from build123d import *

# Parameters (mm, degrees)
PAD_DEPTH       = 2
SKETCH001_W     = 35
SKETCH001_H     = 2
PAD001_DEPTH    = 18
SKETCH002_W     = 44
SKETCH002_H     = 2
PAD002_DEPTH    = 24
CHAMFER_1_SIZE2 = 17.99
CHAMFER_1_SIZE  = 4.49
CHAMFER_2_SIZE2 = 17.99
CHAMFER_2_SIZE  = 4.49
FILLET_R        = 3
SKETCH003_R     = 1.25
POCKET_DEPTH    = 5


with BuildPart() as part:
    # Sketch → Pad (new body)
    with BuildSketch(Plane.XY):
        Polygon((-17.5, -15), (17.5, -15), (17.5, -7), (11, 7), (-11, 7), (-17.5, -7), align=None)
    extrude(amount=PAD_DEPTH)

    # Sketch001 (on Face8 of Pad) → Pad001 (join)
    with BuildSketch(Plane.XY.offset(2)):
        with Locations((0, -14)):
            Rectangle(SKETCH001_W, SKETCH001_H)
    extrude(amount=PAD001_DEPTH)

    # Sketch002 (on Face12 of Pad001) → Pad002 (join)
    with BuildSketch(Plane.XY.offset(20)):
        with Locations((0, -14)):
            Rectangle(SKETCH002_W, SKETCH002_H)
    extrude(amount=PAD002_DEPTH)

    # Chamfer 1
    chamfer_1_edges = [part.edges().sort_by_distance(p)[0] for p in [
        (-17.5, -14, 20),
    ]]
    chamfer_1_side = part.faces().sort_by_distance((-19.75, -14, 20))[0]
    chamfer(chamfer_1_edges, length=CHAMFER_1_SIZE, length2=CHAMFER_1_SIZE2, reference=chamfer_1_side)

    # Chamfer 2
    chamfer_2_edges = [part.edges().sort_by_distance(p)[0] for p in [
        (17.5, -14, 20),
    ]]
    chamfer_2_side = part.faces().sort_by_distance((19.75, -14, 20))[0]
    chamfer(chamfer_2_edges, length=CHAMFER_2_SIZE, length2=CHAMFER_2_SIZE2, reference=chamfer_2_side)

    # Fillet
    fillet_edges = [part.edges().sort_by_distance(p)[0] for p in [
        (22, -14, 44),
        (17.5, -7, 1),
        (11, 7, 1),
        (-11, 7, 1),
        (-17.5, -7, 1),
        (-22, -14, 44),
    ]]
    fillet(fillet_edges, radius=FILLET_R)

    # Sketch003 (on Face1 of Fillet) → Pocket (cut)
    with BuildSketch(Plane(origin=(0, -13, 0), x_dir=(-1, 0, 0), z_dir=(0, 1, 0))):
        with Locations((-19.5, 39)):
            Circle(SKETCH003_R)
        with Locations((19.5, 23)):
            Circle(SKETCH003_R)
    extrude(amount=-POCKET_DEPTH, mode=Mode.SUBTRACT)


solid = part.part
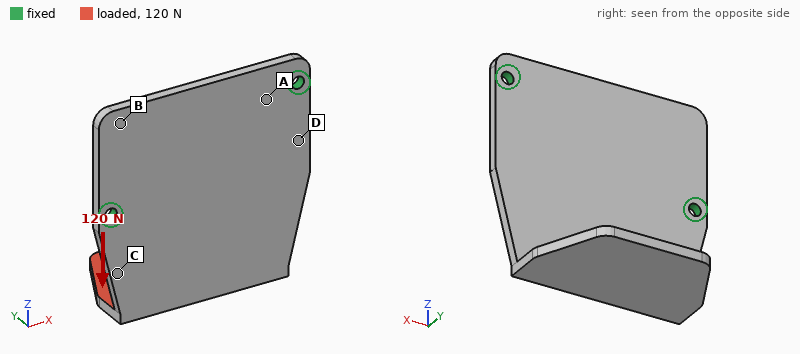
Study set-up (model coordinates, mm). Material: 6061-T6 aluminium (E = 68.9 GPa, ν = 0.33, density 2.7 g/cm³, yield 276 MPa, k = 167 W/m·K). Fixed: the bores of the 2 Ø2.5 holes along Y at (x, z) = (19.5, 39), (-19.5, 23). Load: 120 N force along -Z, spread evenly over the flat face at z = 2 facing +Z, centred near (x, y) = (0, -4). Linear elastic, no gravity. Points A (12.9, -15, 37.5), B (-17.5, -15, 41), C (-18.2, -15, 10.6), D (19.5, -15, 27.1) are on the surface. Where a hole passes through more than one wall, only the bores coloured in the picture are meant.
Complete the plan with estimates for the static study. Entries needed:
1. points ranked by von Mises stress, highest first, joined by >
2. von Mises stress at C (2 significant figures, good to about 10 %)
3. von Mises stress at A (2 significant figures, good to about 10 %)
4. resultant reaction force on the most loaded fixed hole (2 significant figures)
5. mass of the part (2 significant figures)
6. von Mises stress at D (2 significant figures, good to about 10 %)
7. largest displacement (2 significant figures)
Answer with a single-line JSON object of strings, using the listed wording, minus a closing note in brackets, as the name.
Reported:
{"points ranked by von Mises stress, highest first, joined by >": "C > D > A > B", "von Mises stress at C": "57 MPa", "von Mises stress at A": "20 MPa", "resultant reaction force on the most loaded fixed hole": "65 N", "mass of the part": "13 g", "von Mises stress at D": "28 MPa", "largest displacement": "0.58 mm"}
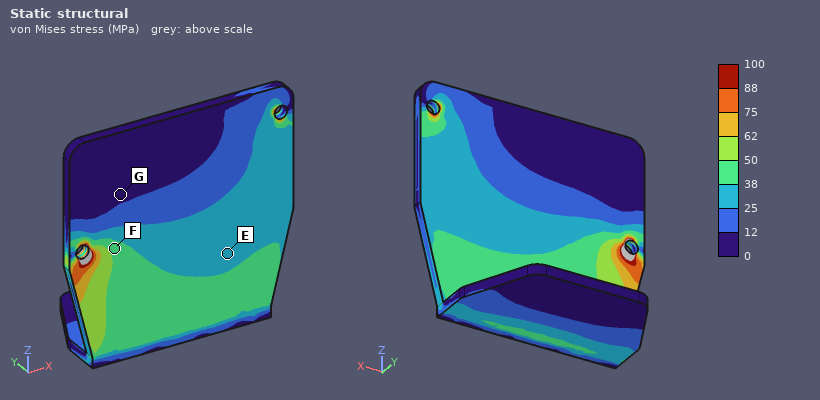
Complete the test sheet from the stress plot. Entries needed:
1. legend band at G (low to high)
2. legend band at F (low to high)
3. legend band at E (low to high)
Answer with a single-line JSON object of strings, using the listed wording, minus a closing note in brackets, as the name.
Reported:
{"legend band at G": "0 to 12 MPa", "legend band at F": "38 to 50 MPa", "legend band at E": "25 to 38 MPa"}
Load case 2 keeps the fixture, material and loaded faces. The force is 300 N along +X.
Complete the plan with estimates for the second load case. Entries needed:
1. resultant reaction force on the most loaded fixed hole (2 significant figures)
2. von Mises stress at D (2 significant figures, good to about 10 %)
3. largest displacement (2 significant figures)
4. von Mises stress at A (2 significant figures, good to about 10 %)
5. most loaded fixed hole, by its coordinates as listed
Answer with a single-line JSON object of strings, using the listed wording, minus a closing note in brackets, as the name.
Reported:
{"resultant reaction force on the most loaded fixed hole": "300 N", "von Mises stress at D": "79 MPa", "largest displacement": "0.74 mm", "von Mises stress at A": "58 MPa", "most loaded fixed hole, by its coordinates as listed": "(-19.5, 23)"}
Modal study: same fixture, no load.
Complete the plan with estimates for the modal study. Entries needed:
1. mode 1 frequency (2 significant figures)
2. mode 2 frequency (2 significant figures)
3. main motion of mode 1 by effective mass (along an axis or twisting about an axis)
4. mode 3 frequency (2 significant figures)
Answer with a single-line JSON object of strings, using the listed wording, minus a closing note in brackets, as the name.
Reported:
{"mode 1 frequency": "850 Hz", "mode 2 frequency": "2100 Hz", "main motion of mode 1 by effective mass": "along Y", "mode 3 frequency": "3100 Hz"}
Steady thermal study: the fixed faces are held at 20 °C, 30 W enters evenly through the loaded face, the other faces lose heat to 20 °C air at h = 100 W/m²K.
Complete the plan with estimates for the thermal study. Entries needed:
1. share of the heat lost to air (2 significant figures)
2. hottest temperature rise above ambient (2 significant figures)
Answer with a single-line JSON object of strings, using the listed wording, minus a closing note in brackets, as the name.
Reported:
{"share of the heat lost to air": "45 %", "hottest temperature rise above ambient": "74 K"}
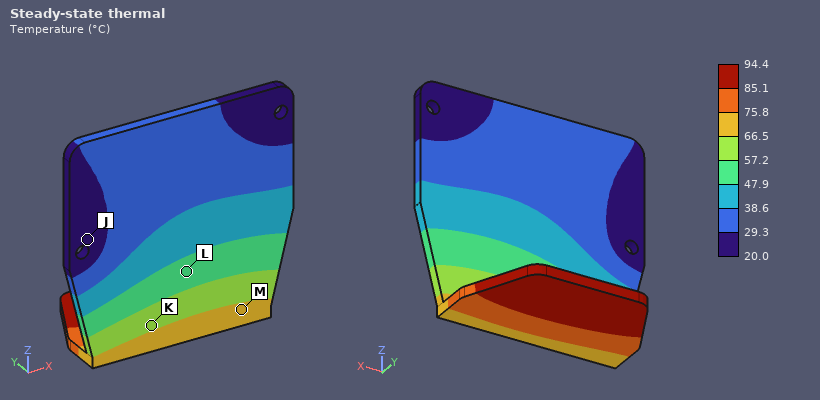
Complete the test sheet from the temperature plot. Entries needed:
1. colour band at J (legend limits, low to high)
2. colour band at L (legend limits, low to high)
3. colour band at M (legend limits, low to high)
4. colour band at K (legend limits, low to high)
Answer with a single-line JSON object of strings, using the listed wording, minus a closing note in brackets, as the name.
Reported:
{"colour band at J": "20.0 to 29.3 °C", "colour band at L": "47.9 to 57.2 °C", "colour band at M": "66.5 to 75.8 °C", "colour band at K": "57.2 to 66.5 °C"}
